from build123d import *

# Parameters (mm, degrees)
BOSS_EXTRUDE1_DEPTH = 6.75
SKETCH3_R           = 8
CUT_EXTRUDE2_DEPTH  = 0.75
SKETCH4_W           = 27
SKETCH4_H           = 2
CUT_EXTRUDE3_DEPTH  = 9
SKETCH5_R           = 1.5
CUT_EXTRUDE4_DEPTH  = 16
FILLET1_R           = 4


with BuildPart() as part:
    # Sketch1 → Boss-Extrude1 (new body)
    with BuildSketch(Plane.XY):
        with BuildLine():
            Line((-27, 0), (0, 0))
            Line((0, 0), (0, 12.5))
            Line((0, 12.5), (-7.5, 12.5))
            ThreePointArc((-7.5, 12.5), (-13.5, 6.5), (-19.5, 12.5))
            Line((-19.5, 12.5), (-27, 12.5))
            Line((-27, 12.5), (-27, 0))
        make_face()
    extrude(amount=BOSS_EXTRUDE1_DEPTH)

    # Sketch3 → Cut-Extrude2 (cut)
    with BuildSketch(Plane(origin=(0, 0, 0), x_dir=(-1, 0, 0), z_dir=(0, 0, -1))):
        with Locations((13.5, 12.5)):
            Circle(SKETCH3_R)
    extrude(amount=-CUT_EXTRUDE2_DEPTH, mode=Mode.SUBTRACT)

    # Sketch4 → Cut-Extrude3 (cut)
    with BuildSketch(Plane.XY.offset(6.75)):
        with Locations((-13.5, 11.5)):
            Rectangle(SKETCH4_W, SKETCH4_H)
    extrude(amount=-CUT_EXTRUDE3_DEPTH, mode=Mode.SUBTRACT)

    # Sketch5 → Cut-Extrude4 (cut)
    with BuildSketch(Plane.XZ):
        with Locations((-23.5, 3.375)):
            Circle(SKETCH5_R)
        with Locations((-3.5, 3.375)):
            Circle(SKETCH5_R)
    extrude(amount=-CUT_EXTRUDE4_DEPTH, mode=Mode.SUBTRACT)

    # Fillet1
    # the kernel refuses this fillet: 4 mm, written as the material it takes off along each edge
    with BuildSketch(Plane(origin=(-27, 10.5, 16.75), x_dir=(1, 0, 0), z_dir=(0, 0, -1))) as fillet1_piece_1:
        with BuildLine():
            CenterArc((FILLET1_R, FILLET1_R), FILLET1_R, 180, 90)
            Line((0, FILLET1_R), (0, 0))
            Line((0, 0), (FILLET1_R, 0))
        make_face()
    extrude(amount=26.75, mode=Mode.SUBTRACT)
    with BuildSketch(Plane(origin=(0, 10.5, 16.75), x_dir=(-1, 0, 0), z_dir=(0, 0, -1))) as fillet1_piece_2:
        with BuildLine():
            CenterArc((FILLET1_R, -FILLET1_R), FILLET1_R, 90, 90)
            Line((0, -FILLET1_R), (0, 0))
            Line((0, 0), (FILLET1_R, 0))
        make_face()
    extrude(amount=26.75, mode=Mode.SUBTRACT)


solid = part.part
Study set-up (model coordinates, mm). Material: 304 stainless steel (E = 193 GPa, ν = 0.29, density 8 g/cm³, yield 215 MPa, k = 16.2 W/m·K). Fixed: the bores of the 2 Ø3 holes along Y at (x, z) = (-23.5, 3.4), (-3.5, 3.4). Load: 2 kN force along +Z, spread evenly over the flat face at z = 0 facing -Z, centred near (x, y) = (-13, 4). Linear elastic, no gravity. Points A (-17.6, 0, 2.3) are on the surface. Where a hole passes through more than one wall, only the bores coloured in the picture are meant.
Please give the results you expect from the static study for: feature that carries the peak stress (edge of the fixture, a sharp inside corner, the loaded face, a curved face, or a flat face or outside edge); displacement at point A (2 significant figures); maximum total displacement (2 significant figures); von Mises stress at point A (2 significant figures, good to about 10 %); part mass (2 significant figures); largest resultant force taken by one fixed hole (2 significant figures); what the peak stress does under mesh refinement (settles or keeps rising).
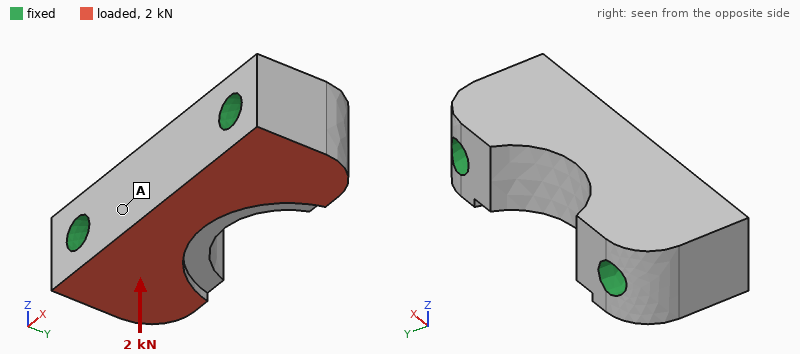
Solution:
edge of the fixture
1.3 µm
1.8 µm
17 MPa
12 g
1.0 kN
keeps rising
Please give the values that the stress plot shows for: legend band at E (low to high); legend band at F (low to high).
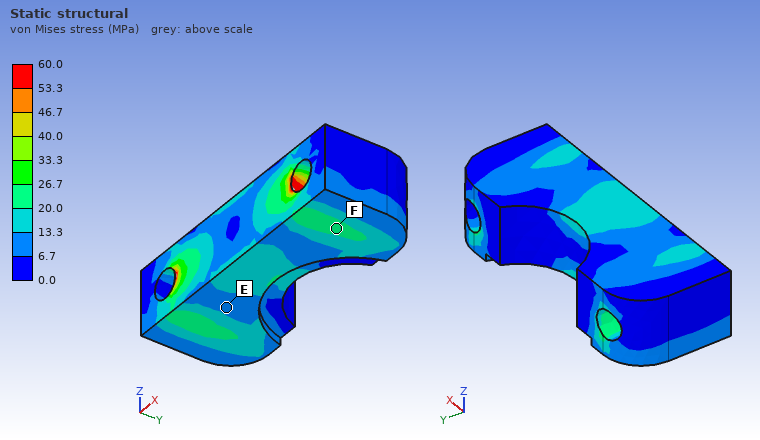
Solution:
6.7 to 13.3 MPa
20.0 to 26.7 MPa
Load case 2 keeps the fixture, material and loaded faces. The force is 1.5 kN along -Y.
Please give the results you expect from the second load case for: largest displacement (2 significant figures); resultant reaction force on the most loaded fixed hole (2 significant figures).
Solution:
1.7 µm
750 N
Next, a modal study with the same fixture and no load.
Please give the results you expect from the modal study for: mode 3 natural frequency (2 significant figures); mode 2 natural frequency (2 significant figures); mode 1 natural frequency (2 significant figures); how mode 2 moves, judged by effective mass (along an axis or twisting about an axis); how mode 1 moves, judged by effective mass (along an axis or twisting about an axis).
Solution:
95 kHz
76 kHz
58 kHz
along Y
along Z
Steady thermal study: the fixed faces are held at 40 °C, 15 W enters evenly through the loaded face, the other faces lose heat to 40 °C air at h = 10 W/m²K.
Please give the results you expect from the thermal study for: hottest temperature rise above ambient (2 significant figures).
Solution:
31 K
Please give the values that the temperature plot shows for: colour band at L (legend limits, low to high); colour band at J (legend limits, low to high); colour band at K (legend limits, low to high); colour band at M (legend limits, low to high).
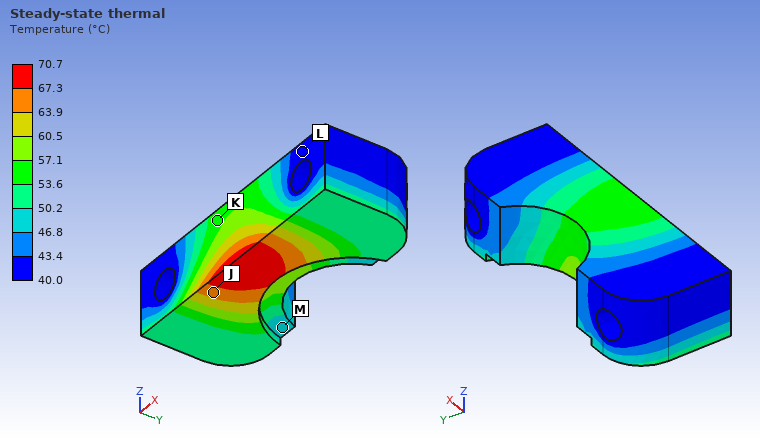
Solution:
40.0 to 43.4 °C
63.9 to 67.3 °C
53.6 to 57.1 °C
46.8 to 50.2 °C
